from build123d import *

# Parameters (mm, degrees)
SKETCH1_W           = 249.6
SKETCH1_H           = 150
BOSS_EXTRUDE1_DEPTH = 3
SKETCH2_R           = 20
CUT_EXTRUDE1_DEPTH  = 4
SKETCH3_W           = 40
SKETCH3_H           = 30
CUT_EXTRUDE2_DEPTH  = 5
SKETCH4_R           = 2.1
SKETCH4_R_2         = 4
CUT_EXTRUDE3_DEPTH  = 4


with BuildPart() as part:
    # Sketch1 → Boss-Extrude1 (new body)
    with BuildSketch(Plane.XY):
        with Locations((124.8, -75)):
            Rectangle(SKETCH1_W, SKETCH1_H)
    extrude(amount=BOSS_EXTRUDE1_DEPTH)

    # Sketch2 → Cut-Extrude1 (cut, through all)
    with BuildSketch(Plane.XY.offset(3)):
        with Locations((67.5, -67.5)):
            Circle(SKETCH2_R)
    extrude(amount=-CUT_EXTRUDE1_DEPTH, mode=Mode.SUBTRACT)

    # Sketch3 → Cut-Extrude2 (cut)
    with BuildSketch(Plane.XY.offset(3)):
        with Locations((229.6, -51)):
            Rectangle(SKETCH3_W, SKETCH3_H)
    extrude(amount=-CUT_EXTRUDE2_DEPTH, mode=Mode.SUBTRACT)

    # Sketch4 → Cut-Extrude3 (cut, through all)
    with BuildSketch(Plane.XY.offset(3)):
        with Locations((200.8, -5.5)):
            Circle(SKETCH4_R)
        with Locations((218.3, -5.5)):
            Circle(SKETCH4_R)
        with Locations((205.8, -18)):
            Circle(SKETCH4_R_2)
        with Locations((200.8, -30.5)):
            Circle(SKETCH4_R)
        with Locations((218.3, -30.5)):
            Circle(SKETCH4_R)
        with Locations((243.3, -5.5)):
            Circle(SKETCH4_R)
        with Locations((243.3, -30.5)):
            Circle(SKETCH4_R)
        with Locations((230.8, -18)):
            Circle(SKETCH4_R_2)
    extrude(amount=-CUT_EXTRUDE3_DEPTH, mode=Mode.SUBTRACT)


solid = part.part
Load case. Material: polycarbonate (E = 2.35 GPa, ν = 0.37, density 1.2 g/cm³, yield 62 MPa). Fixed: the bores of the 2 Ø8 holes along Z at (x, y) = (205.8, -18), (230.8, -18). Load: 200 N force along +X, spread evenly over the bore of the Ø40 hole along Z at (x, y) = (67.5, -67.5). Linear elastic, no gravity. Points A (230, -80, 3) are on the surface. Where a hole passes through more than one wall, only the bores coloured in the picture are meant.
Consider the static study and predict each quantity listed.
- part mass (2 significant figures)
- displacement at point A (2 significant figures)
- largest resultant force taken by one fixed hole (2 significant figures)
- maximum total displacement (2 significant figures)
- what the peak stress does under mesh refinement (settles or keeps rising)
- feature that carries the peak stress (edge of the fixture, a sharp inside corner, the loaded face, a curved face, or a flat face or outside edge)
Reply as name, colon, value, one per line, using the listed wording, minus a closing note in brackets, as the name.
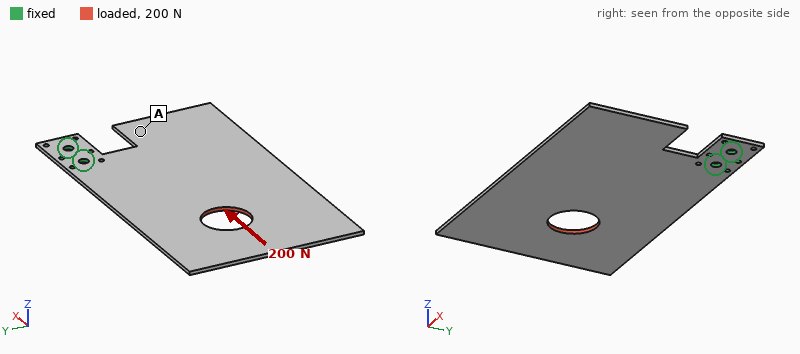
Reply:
part mass: 130 g
displacement at point A: 0.80 mm
largest resultant force taken by one fixed hole: 280 N
maximum total displacement: 2.9 mm
what the peak stress does under mesh refinement: keeps rising
feature that carries the peak stress: a sharp inside corner
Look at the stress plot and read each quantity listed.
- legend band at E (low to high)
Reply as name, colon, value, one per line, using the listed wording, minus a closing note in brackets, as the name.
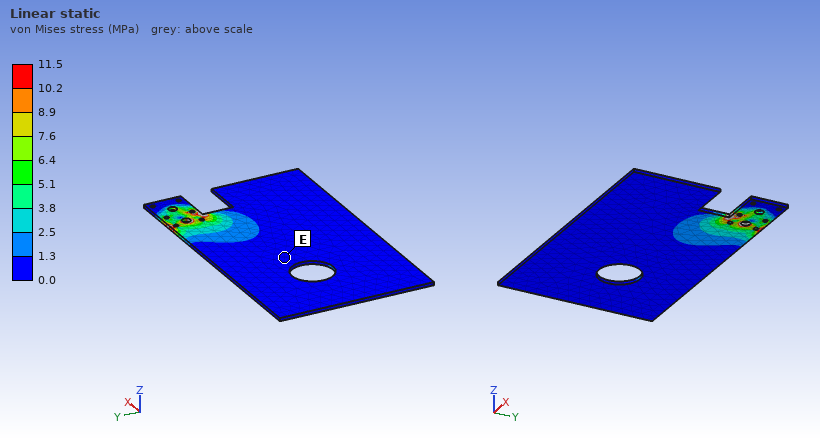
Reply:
legend band at E: 0.0 to 1.3 MPa
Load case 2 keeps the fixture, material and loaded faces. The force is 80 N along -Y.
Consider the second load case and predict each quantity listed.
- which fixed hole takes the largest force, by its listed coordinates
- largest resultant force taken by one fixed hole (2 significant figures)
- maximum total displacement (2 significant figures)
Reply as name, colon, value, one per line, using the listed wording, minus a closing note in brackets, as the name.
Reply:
which fixed hole takes the largest force, by its listed coordinates: (205.8, -18)
largest resultant force taken by one fixed hole: 360 N
maximum total displacement: 3.3 mm
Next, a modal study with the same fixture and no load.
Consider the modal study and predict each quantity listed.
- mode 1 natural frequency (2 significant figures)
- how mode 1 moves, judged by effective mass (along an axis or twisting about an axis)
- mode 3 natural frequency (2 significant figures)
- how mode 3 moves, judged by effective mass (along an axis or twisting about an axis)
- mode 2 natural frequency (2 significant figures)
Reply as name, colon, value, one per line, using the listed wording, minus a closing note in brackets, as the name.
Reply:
mode 1 natural frequency: 11 Hz
how mode 1 moves, judged by effective mass: along Z
mode 3 natural frequency: 57 Hz
how mode 3 moves, judged by effective mass: along Z
mode 2 natural frequency: 23 Hz
